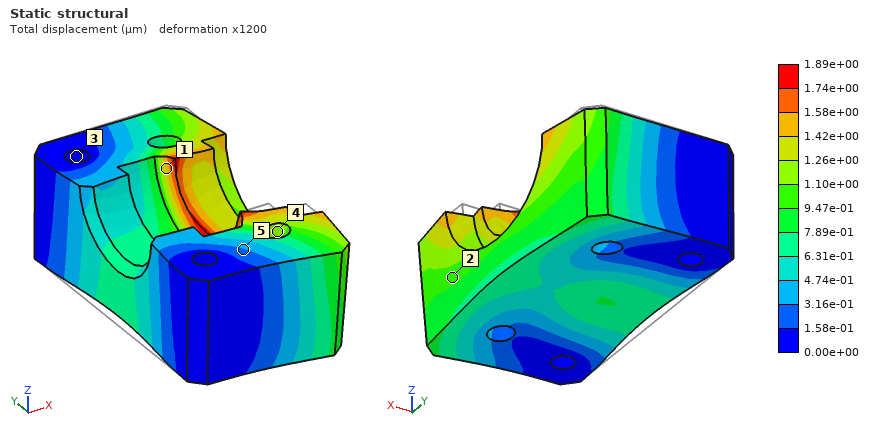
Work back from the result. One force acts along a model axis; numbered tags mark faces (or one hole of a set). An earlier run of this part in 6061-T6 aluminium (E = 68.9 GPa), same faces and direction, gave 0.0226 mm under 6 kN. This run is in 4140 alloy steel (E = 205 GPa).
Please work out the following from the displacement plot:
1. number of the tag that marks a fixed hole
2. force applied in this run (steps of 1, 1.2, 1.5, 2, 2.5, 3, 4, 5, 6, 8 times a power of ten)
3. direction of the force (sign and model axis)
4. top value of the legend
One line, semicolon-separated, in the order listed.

3; 1.5 kN; +X; 1.89e+00 µm
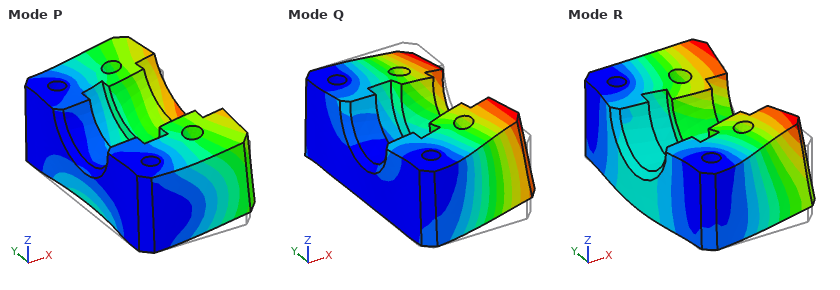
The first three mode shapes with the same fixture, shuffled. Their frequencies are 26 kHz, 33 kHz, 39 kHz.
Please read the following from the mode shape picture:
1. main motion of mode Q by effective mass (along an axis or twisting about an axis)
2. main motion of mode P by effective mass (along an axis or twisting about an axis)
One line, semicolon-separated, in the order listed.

along Y; along Z
